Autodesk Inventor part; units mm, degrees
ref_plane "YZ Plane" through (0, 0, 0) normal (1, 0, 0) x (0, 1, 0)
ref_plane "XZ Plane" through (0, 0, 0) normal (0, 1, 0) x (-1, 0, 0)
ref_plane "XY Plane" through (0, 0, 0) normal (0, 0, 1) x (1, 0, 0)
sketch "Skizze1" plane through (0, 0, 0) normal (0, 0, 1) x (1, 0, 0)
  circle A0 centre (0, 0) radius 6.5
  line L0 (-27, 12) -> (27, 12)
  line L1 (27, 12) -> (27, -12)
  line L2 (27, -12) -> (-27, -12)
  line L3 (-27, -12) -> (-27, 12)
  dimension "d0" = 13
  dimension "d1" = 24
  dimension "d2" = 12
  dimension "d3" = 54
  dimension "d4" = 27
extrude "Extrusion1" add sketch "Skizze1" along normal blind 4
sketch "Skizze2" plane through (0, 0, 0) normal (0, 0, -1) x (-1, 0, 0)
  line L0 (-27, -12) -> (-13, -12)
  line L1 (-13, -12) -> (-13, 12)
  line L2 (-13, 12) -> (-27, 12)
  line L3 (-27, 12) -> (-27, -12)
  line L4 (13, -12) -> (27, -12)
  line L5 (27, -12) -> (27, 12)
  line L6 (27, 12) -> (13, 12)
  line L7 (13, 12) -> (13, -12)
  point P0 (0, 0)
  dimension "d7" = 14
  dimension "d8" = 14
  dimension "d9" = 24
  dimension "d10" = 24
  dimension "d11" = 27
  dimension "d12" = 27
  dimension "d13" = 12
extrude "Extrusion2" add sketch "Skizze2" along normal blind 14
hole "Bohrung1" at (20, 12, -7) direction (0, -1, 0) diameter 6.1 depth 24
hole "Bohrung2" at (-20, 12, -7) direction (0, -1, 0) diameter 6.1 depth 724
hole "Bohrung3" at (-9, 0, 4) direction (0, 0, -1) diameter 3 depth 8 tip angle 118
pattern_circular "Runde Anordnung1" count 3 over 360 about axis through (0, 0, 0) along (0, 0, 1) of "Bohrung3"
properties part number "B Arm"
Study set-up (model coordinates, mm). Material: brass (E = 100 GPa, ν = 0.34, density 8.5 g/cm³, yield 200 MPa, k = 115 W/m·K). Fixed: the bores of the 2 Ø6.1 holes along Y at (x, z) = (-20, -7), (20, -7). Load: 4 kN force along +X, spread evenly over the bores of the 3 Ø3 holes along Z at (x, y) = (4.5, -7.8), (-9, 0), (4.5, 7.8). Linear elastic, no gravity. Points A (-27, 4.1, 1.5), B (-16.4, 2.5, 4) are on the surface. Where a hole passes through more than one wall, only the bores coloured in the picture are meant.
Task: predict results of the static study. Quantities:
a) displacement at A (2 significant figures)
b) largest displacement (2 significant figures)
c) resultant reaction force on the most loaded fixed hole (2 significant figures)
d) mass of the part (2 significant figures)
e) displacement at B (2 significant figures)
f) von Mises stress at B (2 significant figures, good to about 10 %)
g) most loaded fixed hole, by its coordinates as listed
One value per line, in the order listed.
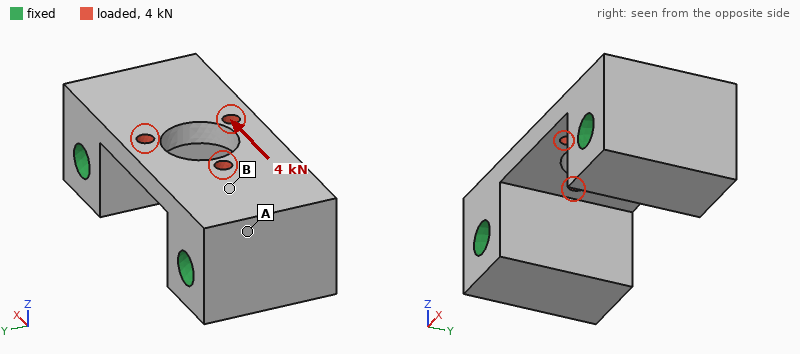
2.5 µm
8.8 µm
2.1 kN
110 g
3.8 µm
23 MPa
(-20, -7)
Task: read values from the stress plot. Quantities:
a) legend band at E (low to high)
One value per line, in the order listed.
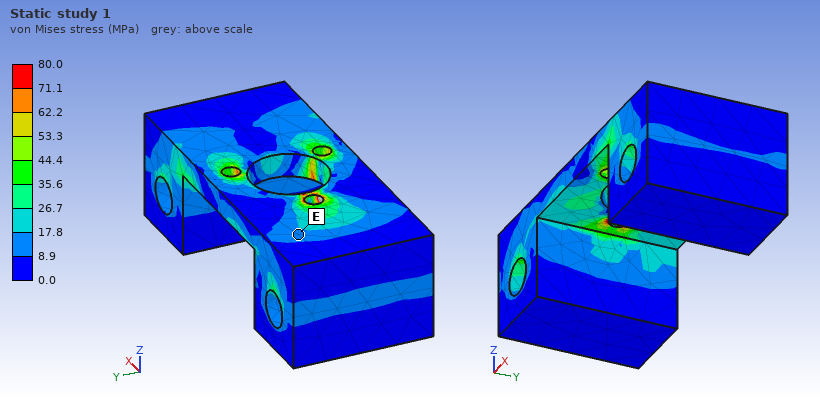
8.9 to 17.8 MPa
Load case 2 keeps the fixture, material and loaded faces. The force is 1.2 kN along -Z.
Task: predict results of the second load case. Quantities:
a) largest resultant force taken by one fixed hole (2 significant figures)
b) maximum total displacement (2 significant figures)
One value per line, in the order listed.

690 N
16 µm
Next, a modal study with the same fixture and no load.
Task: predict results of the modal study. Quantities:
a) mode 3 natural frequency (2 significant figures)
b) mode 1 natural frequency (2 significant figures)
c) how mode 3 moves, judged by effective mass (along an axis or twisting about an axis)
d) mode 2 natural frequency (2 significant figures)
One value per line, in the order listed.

24 kHz
15 kHz
along X
17 kHz
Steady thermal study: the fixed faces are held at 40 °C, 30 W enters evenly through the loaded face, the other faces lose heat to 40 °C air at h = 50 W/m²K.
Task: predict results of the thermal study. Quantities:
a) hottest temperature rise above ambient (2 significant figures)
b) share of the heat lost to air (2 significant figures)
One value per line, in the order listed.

23 K
3.5 %
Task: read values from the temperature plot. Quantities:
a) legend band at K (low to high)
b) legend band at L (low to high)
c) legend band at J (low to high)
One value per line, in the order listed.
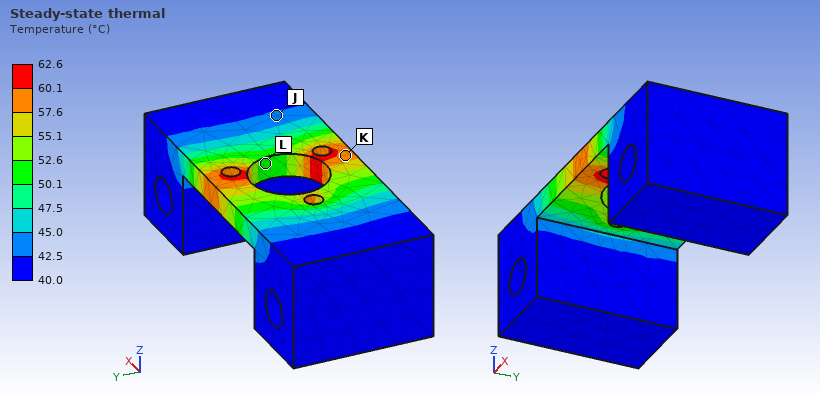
57.6 to 60.1 °C
50.1 to 52.6 °C
42.5 to 45.0 °C
